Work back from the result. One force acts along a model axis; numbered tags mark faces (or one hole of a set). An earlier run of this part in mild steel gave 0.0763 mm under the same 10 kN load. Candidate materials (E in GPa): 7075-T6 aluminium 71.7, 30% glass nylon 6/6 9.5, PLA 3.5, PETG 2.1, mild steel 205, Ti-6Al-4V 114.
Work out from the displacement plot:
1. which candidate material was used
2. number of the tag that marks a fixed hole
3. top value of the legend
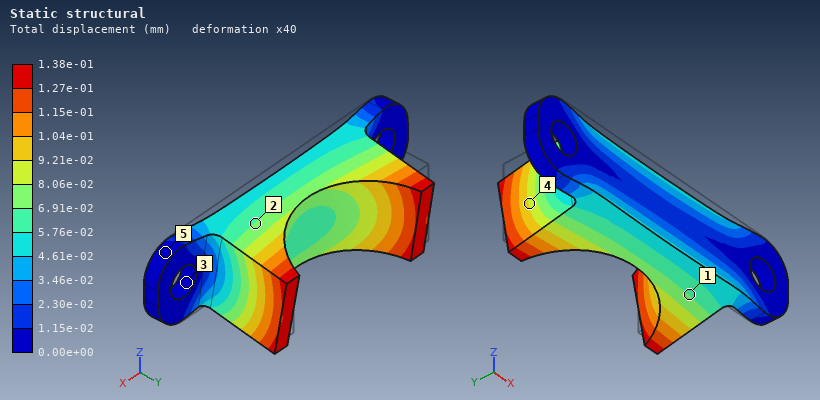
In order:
Ti-6Al-4V
3
1.38e-01 mm
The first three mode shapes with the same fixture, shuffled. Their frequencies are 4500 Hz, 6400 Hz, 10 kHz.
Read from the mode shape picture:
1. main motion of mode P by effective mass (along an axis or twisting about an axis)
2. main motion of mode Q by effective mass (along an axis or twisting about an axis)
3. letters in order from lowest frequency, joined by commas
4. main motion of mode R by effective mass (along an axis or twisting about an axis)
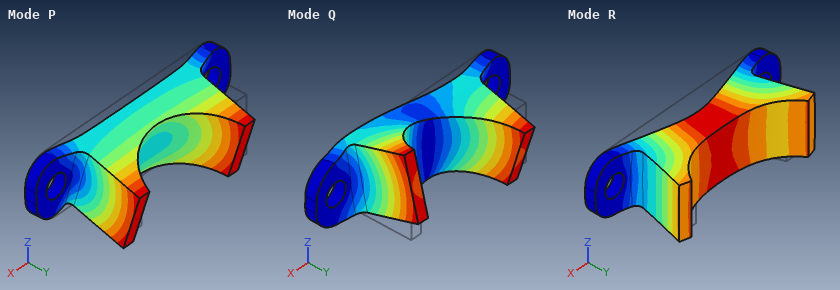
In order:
along Z
twisting about Y
P, R, Q
along Y
